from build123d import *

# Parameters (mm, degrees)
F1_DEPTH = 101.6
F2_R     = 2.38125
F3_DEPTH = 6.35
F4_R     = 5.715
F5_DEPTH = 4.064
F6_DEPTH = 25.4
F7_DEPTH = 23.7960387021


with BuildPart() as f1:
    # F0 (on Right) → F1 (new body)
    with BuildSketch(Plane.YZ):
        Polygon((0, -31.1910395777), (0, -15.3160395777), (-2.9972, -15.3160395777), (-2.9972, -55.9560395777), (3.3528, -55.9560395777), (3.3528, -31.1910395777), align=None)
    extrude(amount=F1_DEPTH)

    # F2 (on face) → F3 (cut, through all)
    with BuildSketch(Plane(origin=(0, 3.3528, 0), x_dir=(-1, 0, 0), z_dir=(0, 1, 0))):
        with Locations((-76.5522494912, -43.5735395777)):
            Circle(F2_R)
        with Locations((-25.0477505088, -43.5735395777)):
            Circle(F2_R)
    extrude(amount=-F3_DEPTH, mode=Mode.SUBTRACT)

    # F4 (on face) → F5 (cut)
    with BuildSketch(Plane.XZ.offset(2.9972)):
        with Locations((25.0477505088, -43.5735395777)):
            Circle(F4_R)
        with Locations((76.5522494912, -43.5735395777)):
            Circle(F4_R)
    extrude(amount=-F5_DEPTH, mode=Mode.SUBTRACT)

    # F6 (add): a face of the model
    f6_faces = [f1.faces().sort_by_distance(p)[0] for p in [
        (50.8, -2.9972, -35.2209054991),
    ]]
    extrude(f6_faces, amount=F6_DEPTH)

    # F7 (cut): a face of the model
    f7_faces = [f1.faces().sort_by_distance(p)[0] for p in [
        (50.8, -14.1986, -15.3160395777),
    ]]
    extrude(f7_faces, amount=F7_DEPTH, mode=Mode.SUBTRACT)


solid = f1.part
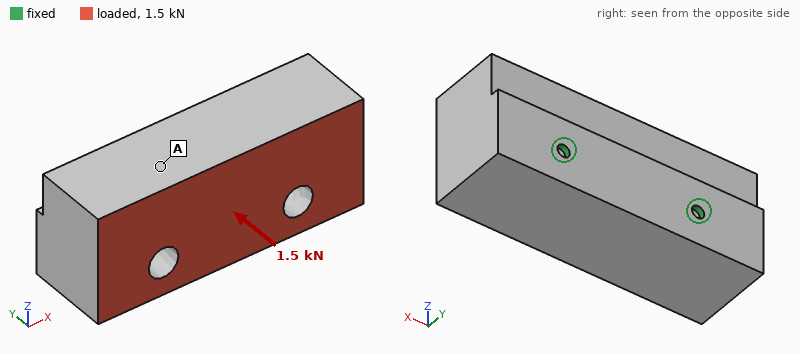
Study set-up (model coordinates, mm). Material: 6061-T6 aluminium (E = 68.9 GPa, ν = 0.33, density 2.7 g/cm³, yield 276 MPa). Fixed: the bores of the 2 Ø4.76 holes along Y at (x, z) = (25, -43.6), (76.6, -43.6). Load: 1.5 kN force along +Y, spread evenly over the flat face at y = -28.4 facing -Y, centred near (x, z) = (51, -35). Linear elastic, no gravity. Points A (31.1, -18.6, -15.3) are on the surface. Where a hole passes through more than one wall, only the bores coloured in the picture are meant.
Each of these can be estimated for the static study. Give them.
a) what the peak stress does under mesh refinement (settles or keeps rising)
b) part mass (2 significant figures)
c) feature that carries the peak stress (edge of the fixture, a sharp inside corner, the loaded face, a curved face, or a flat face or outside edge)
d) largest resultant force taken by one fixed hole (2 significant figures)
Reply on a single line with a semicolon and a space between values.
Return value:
keeps rising; 320 g; edge of the fixture; 750 N
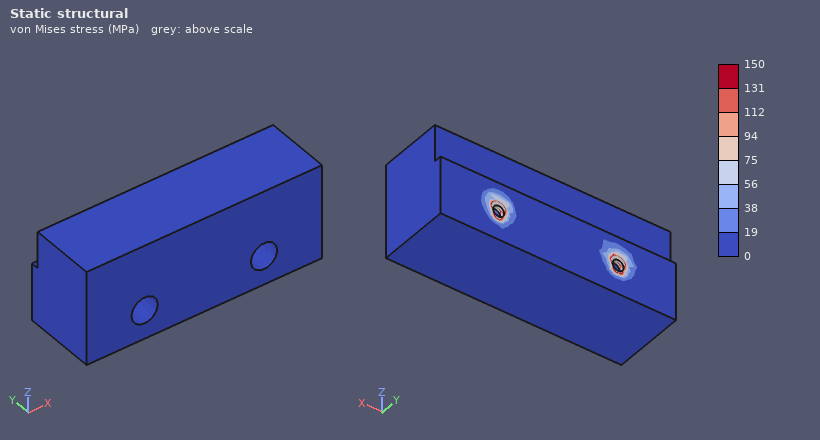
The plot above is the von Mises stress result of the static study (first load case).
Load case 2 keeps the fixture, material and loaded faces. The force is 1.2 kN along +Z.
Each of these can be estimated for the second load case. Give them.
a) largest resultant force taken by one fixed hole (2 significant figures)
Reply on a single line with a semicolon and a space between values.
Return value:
600 N
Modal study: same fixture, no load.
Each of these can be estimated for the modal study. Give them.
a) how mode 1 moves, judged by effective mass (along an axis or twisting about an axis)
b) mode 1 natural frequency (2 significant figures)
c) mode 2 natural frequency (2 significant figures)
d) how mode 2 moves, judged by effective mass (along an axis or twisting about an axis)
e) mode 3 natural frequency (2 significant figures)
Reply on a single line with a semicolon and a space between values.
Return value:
along Z; 730 Hz; 3500 Hz; along X; 4800 Hz
